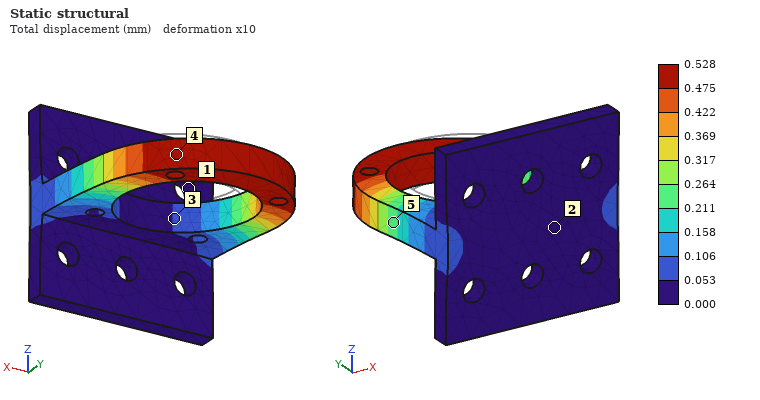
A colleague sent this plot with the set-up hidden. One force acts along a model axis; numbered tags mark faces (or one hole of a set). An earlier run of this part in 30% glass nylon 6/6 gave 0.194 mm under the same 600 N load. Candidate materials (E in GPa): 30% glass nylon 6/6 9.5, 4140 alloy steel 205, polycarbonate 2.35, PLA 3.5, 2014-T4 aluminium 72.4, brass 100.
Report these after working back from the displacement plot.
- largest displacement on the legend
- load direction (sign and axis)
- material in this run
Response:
0.528 mm
-X
PLA
